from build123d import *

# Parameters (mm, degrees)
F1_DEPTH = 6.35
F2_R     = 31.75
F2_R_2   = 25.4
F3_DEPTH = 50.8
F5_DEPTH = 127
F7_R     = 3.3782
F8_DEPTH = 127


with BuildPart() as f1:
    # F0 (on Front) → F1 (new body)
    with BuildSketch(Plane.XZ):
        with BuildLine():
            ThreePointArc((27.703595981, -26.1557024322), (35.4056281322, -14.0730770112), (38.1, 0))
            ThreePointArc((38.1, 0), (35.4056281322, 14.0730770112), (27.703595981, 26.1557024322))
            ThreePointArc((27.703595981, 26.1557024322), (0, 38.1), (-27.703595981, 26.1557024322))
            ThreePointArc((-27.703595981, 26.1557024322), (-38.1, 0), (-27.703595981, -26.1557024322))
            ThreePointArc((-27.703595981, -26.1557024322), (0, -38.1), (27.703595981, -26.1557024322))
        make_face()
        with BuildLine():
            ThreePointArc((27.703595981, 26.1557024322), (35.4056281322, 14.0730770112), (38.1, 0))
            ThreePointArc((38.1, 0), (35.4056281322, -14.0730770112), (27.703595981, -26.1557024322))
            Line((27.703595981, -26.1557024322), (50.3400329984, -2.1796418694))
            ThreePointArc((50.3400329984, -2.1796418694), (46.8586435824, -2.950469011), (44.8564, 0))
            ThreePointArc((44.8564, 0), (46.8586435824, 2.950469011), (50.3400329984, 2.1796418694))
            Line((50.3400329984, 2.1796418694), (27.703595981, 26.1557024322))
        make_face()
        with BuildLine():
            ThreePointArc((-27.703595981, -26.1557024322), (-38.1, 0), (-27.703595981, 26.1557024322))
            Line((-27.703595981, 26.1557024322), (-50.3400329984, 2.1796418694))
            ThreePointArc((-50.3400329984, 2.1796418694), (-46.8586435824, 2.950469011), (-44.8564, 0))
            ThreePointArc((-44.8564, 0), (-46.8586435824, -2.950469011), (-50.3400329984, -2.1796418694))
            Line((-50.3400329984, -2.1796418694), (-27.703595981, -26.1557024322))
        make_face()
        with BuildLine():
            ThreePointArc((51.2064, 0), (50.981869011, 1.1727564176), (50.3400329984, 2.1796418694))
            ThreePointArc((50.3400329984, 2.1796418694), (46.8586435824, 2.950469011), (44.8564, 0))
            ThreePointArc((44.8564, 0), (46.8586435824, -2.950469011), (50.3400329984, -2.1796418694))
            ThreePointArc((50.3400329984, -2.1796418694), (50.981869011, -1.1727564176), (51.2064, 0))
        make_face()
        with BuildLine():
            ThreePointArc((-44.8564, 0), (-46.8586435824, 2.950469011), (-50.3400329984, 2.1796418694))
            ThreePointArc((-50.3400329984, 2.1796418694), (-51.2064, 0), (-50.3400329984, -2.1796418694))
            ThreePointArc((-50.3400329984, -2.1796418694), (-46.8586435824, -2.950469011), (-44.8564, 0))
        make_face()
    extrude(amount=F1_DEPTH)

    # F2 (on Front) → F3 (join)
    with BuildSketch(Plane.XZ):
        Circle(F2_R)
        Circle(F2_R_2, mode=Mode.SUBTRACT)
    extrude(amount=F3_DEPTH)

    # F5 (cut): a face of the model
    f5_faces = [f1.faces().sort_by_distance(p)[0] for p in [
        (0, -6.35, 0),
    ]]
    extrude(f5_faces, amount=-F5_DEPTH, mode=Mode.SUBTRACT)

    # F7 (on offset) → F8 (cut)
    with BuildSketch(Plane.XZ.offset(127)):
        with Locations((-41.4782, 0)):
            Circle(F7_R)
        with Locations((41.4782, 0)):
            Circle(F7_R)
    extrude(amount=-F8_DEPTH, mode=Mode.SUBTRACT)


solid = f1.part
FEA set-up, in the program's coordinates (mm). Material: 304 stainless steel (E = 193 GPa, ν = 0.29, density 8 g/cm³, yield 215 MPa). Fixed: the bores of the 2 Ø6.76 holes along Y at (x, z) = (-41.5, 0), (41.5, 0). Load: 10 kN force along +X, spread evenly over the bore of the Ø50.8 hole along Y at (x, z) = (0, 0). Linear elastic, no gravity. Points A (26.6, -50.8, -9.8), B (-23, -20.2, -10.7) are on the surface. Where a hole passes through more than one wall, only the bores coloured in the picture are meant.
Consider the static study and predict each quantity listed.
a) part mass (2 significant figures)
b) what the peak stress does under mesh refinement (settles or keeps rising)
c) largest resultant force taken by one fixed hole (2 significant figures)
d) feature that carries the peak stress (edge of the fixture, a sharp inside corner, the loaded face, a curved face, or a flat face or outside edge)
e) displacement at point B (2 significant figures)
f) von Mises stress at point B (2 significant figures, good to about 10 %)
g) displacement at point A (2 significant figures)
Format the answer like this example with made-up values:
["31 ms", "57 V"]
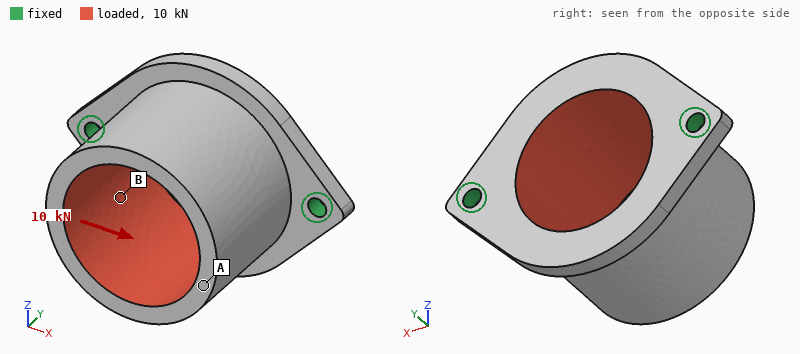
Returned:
["560 g", "keeps rising", "5.9 kN", "edge of the fixture", "12 µm", "24 MPa", "24 µm"]
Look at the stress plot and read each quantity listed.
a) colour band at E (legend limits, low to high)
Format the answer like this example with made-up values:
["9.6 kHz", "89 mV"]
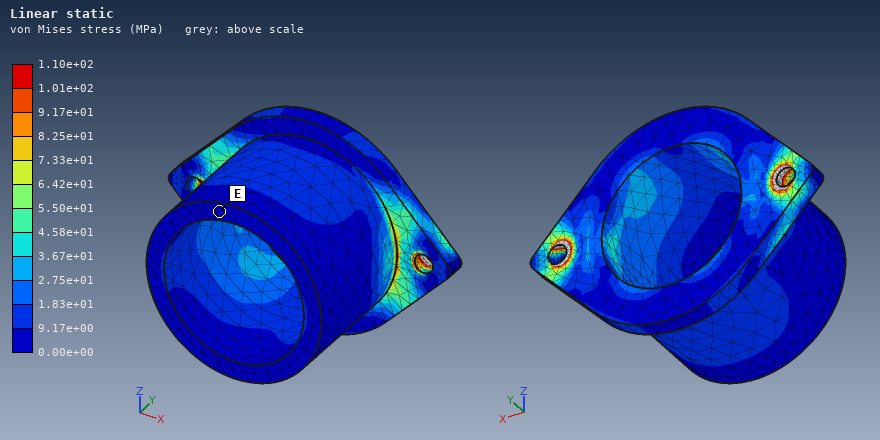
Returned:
["0.00e+00 to 9.17e+00 MPa"]
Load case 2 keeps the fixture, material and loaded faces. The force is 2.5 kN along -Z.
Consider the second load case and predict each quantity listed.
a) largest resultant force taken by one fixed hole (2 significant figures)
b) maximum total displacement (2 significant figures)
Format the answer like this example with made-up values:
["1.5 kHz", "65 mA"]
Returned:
["1.3 kN", "0.10 mm"]
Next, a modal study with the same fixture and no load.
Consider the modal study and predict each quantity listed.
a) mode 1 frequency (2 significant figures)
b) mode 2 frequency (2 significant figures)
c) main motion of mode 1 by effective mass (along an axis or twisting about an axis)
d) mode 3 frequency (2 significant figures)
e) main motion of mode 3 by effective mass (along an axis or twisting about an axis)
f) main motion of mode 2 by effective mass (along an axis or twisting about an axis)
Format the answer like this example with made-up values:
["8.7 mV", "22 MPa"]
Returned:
["1200 Hz", "4000 Hz", "along Z", "5100 Hz", "along X", "along Y"]
